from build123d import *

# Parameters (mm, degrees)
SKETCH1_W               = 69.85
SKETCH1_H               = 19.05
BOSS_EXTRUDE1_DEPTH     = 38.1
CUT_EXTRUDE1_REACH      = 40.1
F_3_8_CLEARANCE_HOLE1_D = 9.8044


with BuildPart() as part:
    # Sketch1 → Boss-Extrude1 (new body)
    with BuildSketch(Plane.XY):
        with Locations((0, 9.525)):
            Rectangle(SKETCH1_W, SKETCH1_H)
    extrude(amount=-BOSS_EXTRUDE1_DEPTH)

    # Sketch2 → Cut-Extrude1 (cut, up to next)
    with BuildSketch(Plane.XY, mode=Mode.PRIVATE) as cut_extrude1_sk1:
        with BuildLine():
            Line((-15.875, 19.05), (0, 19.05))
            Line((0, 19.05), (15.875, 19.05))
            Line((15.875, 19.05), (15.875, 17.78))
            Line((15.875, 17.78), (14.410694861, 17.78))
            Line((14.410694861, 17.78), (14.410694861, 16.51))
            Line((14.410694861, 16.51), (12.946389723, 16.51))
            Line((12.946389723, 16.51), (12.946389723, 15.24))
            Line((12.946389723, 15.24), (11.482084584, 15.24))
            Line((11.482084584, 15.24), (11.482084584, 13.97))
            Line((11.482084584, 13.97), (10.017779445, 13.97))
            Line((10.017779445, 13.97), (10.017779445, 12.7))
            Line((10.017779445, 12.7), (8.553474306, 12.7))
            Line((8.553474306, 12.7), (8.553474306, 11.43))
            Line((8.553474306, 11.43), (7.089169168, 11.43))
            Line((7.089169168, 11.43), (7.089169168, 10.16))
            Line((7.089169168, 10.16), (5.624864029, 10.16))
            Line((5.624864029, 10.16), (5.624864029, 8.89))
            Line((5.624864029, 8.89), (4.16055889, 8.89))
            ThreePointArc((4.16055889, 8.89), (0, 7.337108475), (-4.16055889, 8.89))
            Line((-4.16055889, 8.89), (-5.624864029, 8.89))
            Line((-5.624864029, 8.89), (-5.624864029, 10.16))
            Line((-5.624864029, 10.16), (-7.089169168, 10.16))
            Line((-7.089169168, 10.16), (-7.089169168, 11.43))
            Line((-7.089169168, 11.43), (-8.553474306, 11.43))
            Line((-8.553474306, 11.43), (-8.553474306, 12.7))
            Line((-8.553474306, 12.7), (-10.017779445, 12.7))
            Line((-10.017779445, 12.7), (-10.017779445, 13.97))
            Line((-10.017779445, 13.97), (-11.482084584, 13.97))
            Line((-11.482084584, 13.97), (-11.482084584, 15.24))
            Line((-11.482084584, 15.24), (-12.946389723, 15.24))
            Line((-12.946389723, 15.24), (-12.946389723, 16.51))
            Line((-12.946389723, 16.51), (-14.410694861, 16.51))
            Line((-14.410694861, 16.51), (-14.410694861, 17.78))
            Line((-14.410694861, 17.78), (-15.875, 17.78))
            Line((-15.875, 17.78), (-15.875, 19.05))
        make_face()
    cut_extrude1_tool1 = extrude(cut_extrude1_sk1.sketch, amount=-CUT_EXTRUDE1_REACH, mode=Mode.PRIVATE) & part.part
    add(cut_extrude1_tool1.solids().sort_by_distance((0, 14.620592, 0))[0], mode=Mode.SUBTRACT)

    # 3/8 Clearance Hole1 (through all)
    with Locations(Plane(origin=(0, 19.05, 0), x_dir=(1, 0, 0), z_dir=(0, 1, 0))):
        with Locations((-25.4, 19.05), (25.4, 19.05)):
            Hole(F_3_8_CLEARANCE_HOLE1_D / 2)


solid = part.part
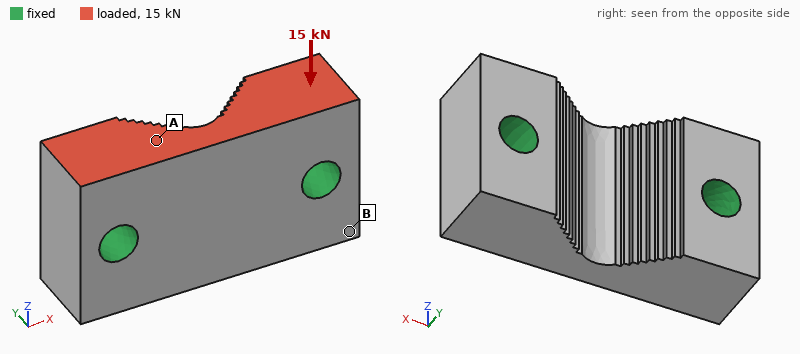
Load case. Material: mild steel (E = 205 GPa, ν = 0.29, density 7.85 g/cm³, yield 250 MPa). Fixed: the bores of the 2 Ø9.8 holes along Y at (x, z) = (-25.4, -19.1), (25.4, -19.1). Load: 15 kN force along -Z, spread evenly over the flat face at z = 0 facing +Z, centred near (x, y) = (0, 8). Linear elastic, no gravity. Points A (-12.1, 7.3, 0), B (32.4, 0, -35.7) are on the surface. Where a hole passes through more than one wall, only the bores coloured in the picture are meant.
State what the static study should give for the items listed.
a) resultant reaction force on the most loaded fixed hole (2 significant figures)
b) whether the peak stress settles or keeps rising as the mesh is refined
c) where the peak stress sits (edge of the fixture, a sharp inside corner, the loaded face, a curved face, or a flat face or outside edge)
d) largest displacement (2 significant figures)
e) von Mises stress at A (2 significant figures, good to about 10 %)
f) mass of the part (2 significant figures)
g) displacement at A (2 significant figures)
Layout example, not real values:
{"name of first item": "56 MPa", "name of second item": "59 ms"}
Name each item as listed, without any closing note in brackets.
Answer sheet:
{"resultant reaction force on the most loaded fixed hole": "7.5 kN", "whether the peak stress settles or keeps rising as the mesh is refined": "keeps rising", "where the peak stress sits": "edge of the fixture", "largest displacement": "3.2 µm", "von Mises stress at A": "12 MPa", "mass of the part": "310 g", "displacement at A": "2.2 µm"}
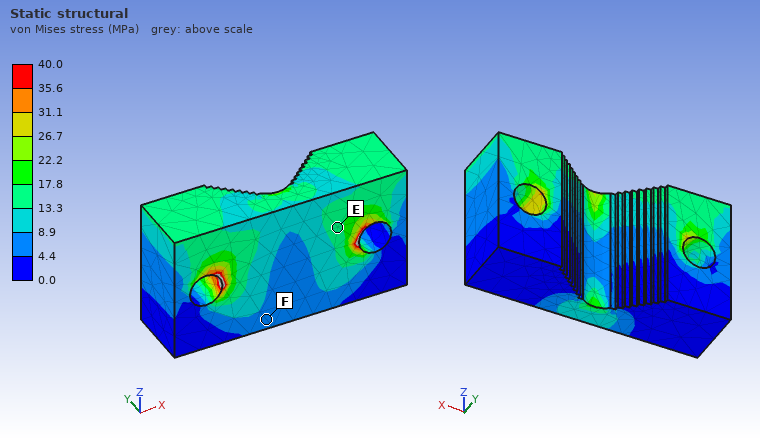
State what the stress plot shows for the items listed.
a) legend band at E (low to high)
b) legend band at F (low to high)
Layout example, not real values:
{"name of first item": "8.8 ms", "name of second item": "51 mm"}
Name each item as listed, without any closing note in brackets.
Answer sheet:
{"legend band at E": "13.3 to 17.8 MPa", "legend band at F": "4.4 to 8.9 MPa"}
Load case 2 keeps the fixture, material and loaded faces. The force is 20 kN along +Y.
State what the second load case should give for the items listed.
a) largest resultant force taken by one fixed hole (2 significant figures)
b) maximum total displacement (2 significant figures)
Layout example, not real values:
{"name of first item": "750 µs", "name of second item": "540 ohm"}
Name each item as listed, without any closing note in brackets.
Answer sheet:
{"largest resultant force taken by one fixed hole": "10 kN", "maximum total displacement": "19 µm"}
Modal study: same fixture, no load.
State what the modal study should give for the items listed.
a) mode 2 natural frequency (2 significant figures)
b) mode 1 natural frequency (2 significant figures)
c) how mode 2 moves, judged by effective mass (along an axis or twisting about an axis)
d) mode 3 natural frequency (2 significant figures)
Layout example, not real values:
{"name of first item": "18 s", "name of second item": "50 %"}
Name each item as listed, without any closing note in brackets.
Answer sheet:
{"mode 2 natural frequency": "25 kHz", "mode 1 natural frequency": "23 kHz", "how mode 2 moves, judged by effective mass": "along Y", "mode 3 natural frequency": "28 kHz"}
